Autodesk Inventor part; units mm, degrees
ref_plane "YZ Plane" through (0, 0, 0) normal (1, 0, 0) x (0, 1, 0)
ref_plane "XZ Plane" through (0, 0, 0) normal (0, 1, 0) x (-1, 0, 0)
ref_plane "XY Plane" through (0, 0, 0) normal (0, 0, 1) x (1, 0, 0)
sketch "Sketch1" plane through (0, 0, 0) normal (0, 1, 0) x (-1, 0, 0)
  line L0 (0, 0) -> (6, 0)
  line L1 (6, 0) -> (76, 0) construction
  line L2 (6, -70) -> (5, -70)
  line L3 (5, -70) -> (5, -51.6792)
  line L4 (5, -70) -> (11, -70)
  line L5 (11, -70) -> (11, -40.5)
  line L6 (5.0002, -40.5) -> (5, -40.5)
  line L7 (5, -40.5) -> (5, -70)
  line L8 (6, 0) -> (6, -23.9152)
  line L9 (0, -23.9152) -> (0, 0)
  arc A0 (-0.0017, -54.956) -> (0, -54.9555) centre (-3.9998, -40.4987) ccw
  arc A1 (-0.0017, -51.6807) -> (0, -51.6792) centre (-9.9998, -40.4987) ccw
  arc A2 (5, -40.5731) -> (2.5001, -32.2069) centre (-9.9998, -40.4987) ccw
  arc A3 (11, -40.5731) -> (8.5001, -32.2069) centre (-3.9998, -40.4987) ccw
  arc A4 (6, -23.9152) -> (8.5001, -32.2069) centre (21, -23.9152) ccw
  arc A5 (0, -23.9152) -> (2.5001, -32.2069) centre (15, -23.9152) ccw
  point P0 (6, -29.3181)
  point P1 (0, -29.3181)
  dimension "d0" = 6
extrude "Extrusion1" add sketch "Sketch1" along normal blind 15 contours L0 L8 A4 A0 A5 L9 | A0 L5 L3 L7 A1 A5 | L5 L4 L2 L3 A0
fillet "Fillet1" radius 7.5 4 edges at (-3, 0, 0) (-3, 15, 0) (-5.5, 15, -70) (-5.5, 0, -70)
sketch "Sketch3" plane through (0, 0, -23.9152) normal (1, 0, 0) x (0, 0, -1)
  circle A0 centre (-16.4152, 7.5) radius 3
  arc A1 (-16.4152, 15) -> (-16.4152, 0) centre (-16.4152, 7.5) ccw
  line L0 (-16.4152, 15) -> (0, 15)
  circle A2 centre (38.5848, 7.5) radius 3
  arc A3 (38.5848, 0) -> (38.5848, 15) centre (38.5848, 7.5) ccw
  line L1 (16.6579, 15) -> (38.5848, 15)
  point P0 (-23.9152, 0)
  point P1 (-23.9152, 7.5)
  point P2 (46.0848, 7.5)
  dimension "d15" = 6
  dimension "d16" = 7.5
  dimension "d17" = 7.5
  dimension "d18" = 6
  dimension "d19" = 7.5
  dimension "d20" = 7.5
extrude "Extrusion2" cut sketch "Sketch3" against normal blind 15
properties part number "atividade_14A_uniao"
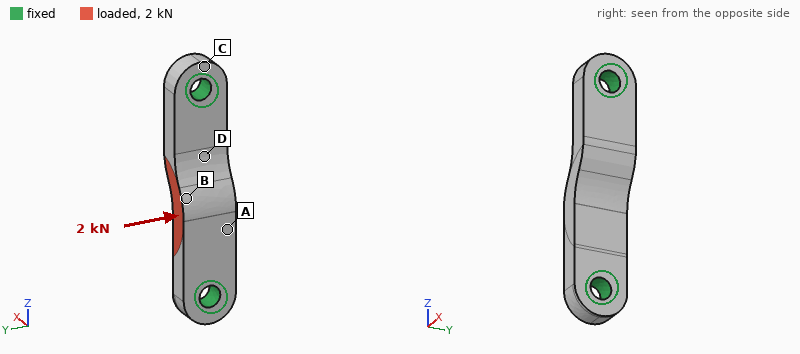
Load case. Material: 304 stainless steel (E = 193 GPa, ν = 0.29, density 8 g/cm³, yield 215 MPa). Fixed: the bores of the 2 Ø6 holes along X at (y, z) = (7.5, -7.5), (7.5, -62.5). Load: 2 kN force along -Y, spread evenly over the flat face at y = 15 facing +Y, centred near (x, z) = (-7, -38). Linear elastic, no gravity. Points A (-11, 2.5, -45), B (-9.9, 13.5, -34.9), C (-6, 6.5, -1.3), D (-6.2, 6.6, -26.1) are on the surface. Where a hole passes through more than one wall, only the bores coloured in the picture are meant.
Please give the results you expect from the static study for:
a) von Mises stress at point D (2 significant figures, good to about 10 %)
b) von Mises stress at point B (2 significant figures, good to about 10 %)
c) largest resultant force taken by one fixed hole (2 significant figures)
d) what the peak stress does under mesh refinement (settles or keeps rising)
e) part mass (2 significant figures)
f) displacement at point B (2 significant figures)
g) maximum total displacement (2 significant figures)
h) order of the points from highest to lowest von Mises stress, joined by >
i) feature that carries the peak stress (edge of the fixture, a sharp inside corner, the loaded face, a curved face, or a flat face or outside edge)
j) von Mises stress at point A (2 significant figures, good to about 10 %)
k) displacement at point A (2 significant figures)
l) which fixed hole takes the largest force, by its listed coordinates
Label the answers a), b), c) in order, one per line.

a) 42 MPa
b) 18 MPa
c) 1.2 kN
d) keeps rising
e) 45 g
f) 12 µm
g) 12 µm
h) D > A > B > C
i) edge of the fixture
j) 27 MPa
k) 9.2 µm
l) (7.5, -62.5)
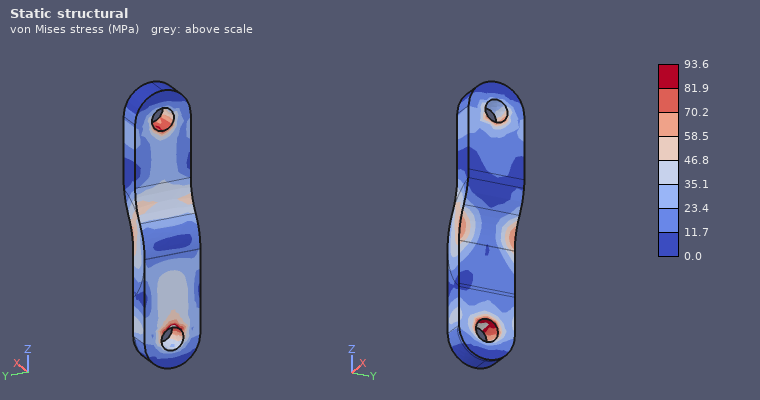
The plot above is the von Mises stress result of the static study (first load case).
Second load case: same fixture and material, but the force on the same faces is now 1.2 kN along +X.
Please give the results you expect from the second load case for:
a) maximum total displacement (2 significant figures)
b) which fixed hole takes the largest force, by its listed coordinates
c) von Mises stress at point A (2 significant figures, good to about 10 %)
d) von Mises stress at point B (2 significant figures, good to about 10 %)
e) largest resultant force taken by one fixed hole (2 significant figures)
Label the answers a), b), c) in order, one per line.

a) 29 µm
b) (7.5, -62.5)
c) 29 MPa
d) 71 MPa
e) 780 N
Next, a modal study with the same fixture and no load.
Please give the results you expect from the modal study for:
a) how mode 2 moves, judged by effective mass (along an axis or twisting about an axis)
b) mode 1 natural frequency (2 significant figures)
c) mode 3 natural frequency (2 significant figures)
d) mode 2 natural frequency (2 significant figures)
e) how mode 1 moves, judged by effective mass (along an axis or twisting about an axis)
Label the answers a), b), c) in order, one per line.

a) along Y
b) 10 kHz
c) 20 kHz
d) 16 kHz
e) along X
